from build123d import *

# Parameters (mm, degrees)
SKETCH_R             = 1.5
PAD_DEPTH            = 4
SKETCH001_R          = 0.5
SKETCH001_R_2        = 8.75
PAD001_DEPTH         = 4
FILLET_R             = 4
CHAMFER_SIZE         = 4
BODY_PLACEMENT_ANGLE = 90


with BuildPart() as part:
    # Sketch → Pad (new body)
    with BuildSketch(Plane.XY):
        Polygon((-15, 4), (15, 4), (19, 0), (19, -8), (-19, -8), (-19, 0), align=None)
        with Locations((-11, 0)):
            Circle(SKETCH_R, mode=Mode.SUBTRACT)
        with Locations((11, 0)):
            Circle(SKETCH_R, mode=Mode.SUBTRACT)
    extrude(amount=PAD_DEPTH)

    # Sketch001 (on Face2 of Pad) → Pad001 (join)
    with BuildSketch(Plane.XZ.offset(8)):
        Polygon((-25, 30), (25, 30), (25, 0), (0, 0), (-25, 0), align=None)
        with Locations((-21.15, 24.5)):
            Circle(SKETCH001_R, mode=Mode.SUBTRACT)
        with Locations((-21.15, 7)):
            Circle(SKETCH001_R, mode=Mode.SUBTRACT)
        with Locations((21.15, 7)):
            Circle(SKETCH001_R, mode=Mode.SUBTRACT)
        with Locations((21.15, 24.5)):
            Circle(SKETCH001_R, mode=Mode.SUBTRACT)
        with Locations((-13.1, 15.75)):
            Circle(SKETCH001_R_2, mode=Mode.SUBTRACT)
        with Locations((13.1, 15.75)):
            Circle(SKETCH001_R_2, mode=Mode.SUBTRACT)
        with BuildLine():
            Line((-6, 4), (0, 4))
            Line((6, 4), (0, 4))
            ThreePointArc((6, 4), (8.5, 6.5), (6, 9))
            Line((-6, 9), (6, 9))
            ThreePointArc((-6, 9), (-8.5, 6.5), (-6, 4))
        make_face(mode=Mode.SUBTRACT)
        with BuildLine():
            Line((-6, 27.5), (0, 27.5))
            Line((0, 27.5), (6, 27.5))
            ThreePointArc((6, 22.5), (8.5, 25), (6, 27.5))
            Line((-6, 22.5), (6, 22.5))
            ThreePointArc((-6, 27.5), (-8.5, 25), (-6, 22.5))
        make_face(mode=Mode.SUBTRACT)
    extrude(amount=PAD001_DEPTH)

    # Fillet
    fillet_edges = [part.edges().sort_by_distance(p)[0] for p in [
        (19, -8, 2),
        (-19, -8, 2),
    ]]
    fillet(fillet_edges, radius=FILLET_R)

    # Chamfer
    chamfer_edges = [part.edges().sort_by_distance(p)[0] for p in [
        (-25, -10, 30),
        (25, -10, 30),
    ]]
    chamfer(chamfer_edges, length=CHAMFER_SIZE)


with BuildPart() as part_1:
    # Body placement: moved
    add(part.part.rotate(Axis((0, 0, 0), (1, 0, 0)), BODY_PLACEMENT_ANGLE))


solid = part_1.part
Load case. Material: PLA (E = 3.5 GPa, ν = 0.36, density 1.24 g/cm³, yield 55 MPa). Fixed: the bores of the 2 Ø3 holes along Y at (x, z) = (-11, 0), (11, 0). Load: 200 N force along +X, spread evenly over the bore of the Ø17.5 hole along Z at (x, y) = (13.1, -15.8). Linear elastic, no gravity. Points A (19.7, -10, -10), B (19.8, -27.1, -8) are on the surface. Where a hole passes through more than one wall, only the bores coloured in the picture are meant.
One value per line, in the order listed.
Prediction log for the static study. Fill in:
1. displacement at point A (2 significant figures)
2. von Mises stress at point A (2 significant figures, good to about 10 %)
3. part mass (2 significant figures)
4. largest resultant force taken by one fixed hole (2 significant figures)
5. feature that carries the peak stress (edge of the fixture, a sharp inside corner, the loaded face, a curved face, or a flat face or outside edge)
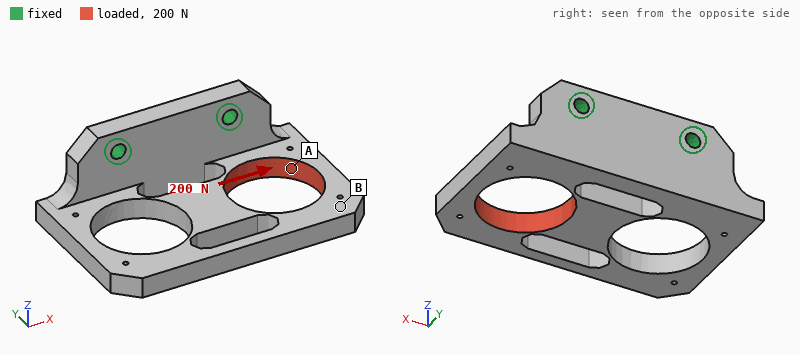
0.28 mm
9.1 MPa
6.3 g
160 N
a flat face or outside edge
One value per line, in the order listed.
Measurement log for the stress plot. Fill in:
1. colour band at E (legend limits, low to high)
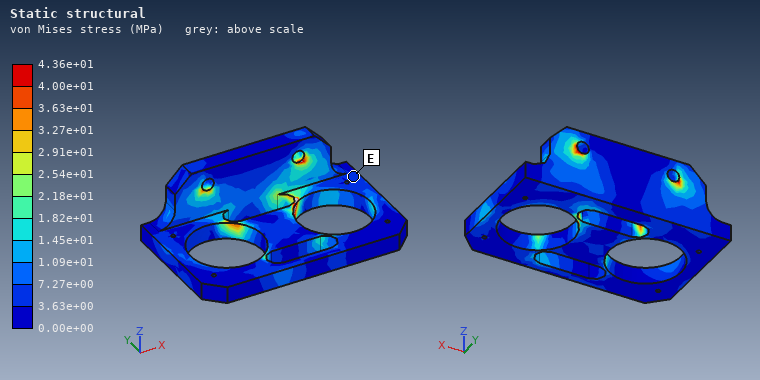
3.63e+00 to 7.27e+00 MPa
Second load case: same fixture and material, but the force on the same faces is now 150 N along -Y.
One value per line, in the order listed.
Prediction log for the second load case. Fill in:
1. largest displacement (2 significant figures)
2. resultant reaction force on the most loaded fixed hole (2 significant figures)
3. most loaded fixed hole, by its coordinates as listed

0.69 mm
150 N
(11, 0)
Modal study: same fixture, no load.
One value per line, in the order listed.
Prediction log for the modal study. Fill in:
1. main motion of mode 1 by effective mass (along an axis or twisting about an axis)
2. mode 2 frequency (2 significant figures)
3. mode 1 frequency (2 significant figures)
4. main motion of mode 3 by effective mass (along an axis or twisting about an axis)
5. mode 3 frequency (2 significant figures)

along Z
1300 Hz
680 Hz
along X
1900 Hz
